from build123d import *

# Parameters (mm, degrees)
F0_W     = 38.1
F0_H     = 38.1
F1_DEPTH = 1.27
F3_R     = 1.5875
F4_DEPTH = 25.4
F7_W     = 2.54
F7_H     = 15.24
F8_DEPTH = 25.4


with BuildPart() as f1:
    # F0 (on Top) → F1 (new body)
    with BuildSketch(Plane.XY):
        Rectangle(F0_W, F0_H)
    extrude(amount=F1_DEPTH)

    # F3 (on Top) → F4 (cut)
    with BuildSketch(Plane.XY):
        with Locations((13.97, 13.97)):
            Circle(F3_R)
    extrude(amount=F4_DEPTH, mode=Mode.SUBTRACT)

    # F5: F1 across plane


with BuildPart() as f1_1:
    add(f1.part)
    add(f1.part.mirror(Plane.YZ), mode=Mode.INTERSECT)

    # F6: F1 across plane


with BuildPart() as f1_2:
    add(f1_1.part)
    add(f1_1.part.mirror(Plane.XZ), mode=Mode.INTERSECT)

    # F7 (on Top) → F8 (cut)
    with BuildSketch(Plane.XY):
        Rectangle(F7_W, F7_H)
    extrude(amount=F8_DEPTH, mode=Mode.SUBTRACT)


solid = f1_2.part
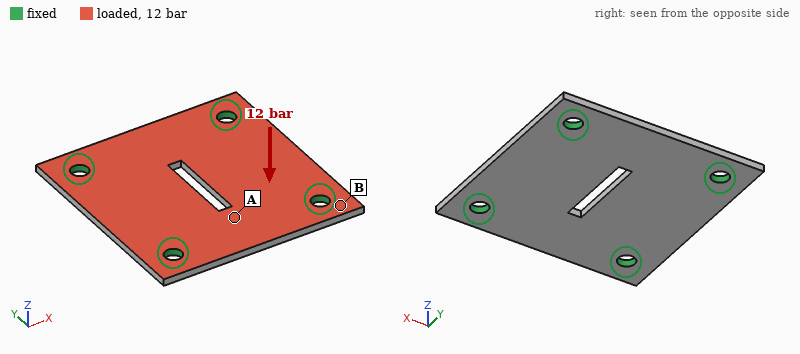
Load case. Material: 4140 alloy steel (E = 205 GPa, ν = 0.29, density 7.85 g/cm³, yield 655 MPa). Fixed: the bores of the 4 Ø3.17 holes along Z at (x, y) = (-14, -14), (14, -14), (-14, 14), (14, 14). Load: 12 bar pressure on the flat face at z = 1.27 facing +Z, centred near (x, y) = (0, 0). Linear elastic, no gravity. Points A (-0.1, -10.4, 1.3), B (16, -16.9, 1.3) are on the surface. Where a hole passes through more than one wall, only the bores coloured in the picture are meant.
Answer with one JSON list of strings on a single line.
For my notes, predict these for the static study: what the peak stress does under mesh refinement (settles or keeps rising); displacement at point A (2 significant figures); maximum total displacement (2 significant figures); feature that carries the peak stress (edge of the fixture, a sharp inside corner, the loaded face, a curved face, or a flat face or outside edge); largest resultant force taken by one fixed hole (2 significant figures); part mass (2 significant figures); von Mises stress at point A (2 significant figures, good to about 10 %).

["keeps rising", "0.081 mm", "0.13 mm", "edge of the fixture", "410 N", "14 g", "210 MPa"]
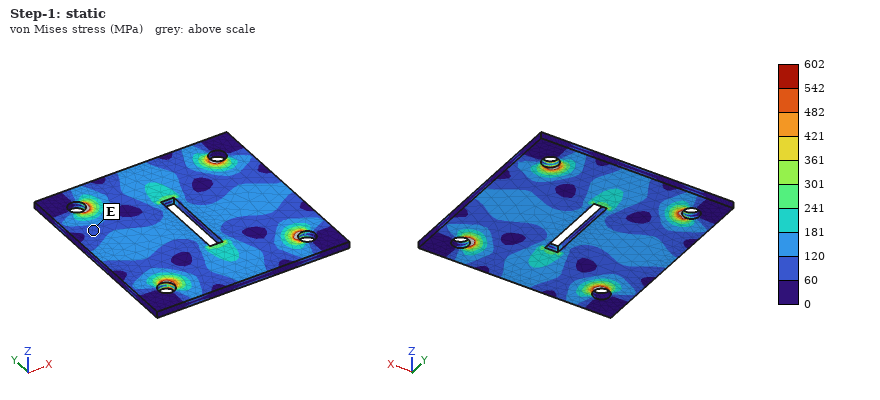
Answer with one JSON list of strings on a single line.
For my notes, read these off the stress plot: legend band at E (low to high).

["60 to 120 MPa"]
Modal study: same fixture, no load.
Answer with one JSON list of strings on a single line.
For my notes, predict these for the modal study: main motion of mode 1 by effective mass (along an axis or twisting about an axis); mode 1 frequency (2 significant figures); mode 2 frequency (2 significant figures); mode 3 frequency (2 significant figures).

["along Z", "6400 Hz", "9800 Hz", "10 kHz"]
